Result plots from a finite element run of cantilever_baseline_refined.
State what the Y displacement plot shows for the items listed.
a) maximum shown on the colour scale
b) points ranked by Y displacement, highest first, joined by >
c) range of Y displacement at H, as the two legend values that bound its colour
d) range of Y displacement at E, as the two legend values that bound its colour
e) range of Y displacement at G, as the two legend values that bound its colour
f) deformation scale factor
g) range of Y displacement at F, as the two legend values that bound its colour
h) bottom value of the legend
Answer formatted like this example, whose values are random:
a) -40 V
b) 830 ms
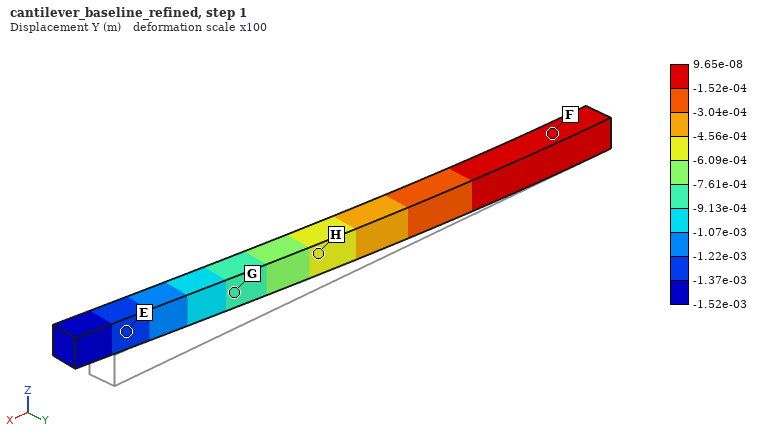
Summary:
a) 9.65e-08 m
b) F > H > G > E
c) -6.09e-04 to -4.56e-04 m
d) -1.37e-03 to -1.22e-03 m
e) -9.13e-04 to -7.61e-04 m
f) 100
g) -1.52e-04 to 9.65e-08 m
h) -1.52e-03 m
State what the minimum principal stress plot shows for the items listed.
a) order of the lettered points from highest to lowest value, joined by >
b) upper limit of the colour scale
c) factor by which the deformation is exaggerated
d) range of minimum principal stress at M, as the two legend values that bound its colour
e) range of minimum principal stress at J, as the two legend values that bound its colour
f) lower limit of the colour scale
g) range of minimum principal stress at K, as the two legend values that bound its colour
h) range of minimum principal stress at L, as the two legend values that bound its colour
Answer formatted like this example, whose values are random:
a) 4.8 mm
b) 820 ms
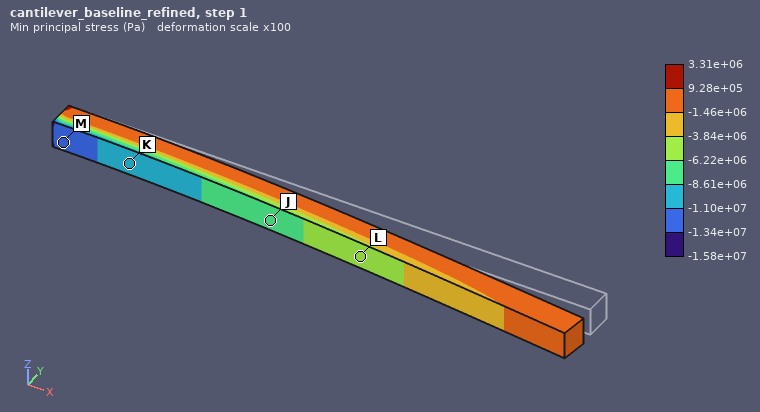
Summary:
a) L > J > K > M
b) 3.31e+06 Pa
c) 100
d) -1.34e+07 to -1.10e+07 Pa
e) -8.61e+06 to -6.22e+06 Pa
f) -1.58e+07 Pa
g) -1.10e+07 to -8.61e+06 Pa
h) -6.22e+06 to -3.84e+06 Pa
